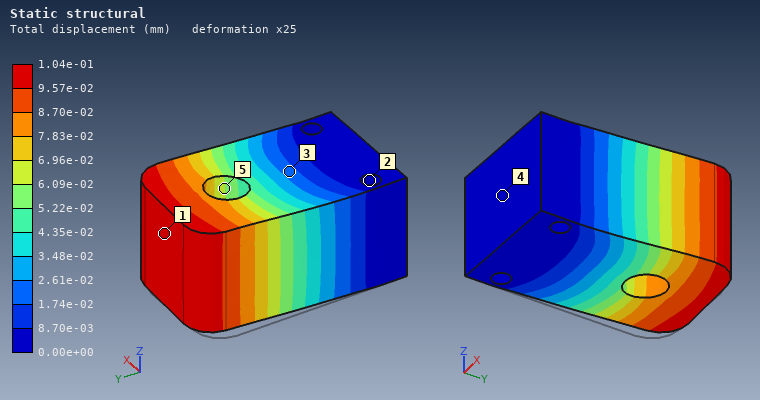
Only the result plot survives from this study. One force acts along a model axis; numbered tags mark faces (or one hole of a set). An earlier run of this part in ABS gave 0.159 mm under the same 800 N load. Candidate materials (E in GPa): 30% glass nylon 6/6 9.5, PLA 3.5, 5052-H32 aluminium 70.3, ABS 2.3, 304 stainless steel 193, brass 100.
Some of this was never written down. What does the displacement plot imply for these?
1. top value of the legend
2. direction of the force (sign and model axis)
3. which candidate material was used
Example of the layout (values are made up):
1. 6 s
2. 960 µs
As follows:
1. 1.04e-01 mm
2. +X
3. PLA
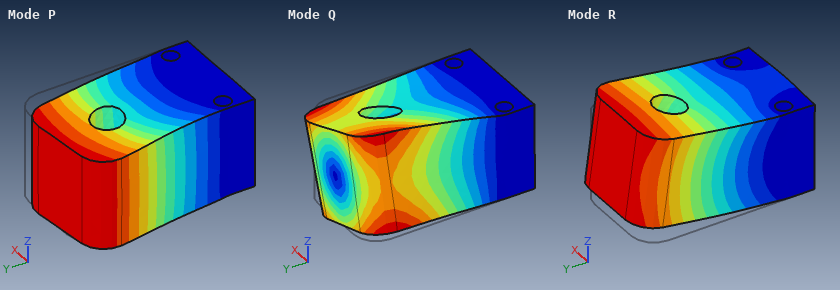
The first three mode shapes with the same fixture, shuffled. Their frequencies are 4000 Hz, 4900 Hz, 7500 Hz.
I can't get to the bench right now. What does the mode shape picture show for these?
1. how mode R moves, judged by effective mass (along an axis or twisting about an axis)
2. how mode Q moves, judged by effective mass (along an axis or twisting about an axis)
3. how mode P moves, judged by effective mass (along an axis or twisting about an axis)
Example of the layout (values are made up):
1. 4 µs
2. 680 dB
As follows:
1. along Z
2. twisting about Y
3. along X
